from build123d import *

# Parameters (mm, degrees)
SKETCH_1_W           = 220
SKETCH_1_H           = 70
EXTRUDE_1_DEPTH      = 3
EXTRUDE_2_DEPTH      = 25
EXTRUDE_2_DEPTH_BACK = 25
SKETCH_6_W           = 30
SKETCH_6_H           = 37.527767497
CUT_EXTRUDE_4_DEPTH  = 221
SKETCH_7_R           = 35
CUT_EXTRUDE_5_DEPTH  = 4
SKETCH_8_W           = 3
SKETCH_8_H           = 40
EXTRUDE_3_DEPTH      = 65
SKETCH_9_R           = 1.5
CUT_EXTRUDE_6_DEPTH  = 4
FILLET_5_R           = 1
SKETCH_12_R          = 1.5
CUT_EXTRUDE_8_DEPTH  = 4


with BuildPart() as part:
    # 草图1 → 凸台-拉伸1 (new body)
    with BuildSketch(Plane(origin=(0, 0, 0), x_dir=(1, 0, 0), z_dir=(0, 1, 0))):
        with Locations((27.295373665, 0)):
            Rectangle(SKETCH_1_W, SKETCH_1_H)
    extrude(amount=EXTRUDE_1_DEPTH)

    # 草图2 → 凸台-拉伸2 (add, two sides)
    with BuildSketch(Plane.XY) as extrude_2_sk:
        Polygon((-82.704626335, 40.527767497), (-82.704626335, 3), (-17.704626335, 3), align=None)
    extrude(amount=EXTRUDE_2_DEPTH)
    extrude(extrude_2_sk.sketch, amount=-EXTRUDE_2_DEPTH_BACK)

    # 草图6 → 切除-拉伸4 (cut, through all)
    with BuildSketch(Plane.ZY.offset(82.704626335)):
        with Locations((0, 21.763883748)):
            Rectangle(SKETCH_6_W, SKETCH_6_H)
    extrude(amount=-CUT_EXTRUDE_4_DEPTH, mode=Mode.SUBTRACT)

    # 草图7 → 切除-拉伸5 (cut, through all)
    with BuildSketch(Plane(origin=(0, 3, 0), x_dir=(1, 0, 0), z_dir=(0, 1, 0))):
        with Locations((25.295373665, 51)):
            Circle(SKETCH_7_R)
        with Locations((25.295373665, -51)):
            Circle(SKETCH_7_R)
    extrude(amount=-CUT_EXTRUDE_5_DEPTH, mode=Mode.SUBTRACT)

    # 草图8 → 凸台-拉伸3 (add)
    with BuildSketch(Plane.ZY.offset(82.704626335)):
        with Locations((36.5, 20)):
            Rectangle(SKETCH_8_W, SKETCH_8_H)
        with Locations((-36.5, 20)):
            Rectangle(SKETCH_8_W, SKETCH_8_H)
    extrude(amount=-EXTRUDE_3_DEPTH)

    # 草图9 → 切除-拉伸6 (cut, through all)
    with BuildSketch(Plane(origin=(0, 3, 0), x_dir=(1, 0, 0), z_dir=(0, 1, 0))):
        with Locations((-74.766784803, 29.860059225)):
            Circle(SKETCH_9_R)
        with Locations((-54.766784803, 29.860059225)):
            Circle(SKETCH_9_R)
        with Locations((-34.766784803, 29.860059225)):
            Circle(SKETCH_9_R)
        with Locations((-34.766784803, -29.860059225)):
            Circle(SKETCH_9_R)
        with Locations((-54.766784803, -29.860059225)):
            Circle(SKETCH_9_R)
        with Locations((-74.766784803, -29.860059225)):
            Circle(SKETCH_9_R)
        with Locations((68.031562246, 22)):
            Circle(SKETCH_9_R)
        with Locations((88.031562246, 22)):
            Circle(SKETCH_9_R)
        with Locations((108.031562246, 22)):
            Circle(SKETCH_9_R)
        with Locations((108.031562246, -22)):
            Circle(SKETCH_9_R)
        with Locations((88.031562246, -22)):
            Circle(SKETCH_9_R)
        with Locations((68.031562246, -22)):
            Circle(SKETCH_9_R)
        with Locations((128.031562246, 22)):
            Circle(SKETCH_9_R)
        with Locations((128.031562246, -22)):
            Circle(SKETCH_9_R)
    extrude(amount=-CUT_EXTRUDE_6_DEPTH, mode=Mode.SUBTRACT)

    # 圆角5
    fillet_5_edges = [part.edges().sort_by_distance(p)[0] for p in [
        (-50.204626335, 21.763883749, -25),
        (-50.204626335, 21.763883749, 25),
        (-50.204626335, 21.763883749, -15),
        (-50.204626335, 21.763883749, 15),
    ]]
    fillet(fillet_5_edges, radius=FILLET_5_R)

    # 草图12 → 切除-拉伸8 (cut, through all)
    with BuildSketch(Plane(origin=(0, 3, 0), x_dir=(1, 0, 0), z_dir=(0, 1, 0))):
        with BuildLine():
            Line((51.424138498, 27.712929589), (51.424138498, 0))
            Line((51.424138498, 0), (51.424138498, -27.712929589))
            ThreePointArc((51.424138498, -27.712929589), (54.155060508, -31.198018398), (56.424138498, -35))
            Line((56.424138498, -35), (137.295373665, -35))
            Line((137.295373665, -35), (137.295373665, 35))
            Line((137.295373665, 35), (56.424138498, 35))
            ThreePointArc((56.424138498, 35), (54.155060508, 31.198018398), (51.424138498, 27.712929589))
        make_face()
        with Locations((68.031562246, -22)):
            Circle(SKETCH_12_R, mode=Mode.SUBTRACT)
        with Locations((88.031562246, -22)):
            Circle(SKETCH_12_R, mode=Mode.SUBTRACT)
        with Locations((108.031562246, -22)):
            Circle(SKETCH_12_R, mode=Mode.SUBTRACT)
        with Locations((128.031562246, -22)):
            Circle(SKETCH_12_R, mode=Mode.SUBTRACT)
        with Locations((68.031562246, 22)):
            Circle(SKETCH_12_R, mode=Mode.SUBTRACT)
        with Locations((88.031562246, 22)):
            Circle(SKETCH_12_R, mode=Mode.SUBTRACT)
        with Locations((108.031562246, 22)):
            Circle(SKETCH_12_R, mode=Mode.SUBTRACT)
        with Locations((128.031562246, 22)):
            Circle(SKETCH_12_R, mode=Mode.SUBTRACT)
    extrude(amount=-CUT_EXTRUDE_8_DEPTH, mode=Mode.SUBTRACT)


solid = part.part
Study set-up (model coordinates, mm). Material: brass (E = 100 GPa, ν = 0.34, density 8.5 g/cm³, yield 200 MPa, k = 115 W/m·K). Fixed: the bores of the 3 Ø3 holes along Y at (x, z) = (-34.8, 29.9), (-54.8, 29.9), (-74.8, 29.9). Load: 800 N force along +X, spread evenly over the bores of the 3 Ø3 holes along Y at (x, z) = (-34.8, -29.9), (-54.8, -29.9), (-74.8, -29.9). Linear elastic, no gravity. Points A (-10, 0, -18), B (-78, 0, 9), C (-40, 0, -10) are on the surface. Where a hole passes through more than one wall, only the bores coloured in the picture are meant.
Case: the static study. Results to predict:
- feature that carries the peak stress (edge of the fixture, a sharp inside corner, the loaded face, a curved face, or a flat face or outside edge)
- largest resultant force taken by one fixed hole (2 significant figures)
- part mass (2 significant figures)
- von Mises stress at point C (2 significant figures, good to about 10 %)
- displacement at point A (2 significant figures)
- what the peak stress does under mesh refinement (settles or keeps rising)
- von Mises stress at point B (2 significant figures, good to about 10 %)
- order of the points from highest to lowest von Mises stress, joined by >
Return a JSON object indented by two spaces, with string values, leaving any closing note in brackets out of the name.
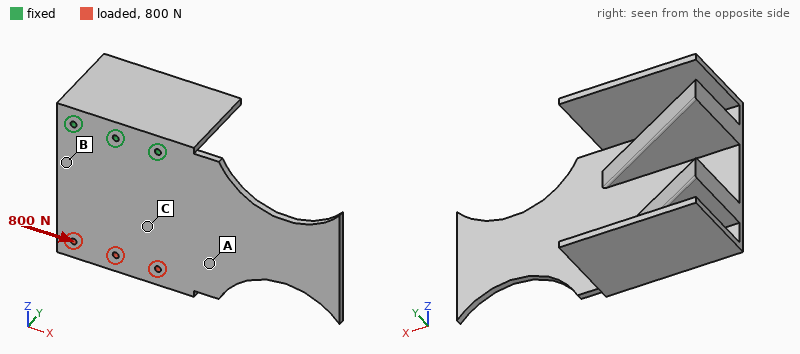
{
  "feature that carries the peak stress": "edge of the fixture",
  "largest resultant force taken by one fixed hole": "1.2 kN",
  "part mass": "540 g",
  "von Mises stress at point C": "9.2 MPa",
  "displacement at point A": "22 µm",
  "what the peak stress does under mesh refinement": "keeps rising",
  "von Mises stress at point B": "13 MPa",
  "order of the points from highest to lowest von Mises stress, joined by >": "B > C > A"
}
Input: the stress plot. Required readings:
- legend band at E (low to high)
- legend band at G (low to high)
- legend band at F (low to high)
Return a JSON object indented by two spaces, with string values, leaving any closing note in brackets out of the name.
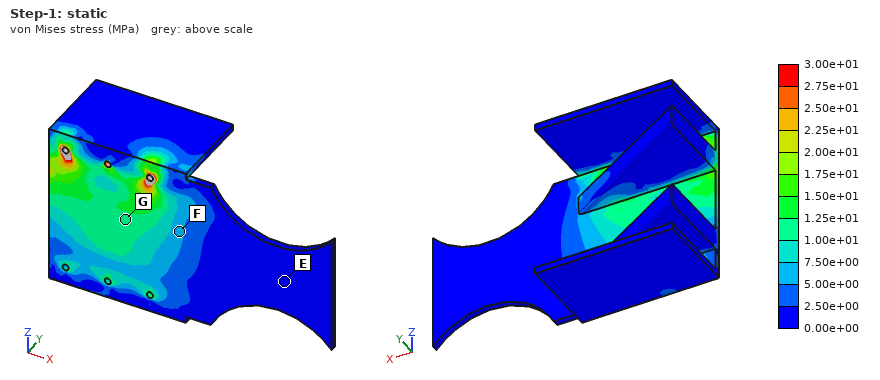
{
  "legend band at E": "0.00e+00 to 2.50e+00 MPa",
  "legend band at G": "1.00e+01 to 1.25e+01 MPa",
  "legend band at F": "5.00e+00 to 7.50e+00 MPa"
}
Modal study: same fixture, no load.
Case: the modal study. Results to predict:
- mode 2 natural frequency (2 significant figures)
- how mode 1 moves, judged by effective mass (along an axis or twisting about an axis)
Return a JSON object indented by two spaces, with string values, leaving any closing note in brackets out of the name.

{
  "mode 2 natural frequency": "310 Hz",
  "how mode 1 moves, judged by effective mass": "along Y"
}
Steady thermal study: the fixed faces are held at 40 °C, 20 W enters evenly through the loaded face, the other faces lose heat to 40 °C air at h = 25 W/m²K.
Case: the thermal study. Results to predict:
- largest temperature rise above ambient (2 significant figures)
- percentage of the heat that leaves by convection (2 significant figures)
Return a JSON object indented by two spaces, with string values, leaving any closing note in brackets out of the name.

{
  "largest temperature rise above ambient": "31 K",
  "percentage of the heat that leaves by convection": "50 %"
}
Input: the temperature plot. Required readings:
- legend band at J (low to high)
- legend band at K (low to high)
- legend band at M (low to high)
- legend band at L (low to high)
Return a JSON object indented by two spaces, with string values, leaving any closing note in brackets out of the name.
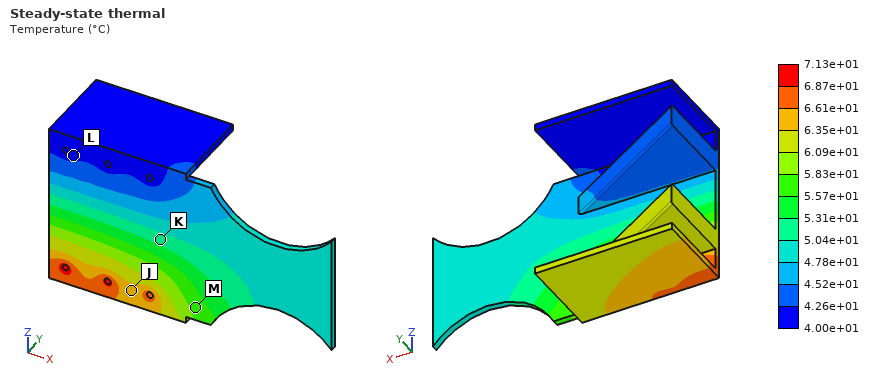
{
  "legend band at J": "6.35e+01 to 6.61e+01 °C",
  "legend band at K": "5.04e+01 to 5.31e+01 °C",
  "legend band at M": "5.57e+01 to 5.83e+01 °C",
  "legend band at L": "4.00e+01 to 4.26e+01 °C"
}
